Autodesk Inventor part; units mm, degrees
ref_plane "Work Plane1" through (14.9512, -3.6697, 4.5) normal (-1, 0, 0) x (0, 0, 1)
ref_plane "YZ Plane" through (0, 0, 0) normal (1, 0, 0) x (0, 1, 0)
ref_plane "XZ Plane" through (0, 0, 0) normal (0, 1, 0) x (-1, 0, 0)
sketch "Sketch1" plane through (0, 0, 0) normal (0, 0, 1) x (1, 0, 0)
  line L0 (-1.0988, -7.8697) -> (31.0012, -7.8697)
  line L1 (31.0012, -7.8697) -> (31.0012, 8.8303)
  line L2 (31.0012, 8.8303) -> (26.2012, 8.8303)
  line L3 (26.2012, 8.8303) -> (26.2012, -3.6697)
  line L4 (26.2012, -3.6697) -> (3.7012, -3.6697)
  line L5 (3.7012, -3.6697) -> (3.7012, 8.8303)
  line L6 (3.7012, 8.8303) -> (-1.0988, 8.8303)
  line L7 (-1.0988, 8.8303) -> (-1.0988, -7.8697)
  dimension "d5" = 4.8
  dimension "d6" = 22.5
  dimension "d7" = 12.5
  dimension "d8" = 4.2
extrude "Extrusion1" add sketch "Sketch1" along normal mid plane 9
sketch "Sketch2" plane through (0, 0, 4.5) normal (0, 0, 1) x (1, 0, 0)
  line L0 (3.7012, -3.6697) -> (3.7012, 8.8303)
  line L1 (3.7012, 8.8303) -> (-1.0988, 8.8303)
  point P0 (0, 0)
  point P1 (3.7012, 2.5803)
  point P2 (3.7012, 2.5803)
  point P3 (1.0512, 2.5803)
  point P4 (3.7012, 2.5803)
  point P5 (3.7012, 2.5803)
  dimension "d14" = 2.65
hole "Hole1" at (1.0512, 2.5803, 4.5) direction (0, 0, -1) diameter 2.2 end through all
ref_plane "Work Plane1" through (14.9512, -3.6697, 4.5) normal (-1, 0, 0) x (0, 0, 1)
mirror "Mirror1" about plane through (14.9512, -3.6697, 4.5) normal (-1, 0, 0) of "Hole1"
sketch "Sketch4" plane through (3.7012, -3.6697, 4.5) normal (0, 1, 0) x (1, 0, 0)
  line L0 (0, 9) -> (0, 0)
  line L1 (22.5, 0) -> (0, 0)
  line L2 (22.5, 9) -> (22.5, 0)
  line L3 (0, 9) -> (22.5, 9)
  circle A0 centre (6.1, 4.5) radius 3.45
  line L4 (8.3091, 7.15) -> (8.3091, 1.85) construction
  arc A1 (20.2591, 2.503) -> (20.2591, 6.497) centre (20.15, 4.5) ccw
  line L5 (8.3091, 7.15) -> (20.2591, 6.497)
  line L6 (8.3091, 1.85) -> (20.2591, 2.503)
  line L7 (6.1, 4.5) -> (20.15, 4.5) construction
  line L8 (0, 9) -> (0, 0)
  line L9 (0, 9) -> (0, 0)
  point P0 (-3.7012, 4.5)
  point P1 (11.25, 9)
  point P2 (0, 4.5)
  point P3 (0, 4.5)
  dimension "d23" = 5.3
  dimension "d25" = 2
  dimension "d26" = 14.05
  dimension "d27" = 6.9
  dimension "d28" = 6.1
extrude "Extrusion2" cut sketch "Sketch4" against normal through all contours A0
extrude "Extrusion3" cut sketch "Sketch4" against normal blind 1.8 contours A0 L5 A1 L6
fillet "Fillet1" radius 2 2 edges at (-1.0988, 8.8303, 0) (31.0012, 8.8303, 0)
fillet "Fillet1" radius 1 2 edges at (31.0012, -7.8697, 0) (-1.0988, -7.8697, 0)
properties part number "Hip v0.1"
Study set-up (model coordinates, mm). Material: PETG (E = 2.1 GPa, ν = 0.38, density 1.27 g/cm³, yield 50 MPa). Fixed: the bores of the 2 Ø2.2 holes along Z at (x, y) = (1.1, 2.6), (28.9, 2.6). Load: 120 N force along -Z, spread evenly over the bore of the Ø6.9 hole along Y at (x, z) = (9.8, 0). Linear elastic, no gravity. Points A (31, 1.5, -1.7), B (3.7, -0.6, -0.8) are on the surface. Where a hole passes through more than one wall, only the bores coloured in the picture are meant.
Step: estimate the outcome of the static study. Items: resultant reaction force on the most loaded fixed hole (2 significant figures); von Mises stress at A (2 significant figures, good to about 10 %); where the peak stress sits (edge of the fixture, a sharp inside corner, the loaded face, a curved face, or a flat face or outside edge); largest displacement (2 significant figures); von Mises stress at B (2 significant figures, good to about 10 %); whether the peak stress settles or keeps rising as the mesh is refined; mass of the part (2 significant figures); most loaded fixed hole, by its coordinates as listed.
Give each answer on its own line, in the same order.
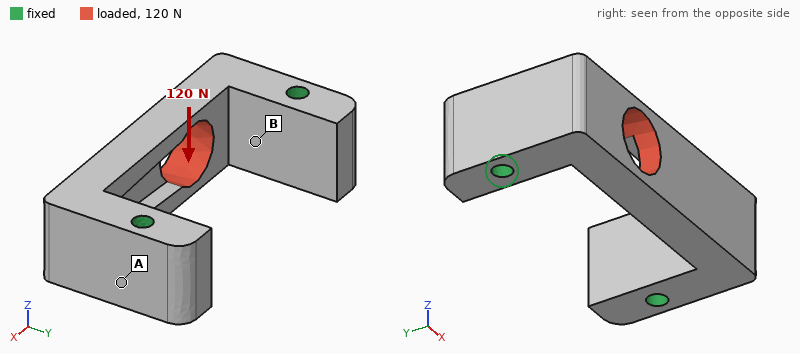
83 N
3.2 MPa
edge of the fixture
0.15 mm
7.7 MPa
keeps rising
2.5 g
(1.1, 2.6)
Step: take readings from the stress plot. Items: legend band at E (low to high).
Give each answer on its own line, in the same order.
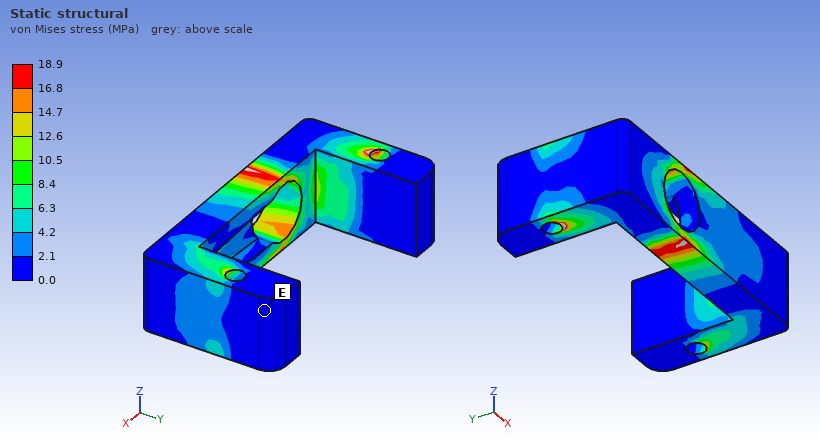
0.0 to 2.1 MPa
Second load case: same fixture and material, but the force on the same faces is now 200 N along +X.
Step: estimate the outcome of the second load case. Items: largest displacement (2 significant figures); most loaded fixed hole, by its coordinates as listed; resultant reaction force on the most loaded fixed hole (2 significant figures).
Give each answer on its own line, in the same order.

0.15 mm
(1.1, 2.6)
110 N
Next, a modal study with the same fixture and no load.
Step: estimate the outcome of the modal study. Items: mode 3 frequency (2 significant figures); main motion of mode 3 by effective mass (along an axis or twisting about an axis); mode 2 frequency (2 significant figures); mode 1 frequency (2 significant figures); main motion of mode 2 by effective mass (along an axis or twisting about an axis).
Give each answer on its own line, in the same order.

6300 Hz
along Y
5800 Hz
5600 Hz
along X
